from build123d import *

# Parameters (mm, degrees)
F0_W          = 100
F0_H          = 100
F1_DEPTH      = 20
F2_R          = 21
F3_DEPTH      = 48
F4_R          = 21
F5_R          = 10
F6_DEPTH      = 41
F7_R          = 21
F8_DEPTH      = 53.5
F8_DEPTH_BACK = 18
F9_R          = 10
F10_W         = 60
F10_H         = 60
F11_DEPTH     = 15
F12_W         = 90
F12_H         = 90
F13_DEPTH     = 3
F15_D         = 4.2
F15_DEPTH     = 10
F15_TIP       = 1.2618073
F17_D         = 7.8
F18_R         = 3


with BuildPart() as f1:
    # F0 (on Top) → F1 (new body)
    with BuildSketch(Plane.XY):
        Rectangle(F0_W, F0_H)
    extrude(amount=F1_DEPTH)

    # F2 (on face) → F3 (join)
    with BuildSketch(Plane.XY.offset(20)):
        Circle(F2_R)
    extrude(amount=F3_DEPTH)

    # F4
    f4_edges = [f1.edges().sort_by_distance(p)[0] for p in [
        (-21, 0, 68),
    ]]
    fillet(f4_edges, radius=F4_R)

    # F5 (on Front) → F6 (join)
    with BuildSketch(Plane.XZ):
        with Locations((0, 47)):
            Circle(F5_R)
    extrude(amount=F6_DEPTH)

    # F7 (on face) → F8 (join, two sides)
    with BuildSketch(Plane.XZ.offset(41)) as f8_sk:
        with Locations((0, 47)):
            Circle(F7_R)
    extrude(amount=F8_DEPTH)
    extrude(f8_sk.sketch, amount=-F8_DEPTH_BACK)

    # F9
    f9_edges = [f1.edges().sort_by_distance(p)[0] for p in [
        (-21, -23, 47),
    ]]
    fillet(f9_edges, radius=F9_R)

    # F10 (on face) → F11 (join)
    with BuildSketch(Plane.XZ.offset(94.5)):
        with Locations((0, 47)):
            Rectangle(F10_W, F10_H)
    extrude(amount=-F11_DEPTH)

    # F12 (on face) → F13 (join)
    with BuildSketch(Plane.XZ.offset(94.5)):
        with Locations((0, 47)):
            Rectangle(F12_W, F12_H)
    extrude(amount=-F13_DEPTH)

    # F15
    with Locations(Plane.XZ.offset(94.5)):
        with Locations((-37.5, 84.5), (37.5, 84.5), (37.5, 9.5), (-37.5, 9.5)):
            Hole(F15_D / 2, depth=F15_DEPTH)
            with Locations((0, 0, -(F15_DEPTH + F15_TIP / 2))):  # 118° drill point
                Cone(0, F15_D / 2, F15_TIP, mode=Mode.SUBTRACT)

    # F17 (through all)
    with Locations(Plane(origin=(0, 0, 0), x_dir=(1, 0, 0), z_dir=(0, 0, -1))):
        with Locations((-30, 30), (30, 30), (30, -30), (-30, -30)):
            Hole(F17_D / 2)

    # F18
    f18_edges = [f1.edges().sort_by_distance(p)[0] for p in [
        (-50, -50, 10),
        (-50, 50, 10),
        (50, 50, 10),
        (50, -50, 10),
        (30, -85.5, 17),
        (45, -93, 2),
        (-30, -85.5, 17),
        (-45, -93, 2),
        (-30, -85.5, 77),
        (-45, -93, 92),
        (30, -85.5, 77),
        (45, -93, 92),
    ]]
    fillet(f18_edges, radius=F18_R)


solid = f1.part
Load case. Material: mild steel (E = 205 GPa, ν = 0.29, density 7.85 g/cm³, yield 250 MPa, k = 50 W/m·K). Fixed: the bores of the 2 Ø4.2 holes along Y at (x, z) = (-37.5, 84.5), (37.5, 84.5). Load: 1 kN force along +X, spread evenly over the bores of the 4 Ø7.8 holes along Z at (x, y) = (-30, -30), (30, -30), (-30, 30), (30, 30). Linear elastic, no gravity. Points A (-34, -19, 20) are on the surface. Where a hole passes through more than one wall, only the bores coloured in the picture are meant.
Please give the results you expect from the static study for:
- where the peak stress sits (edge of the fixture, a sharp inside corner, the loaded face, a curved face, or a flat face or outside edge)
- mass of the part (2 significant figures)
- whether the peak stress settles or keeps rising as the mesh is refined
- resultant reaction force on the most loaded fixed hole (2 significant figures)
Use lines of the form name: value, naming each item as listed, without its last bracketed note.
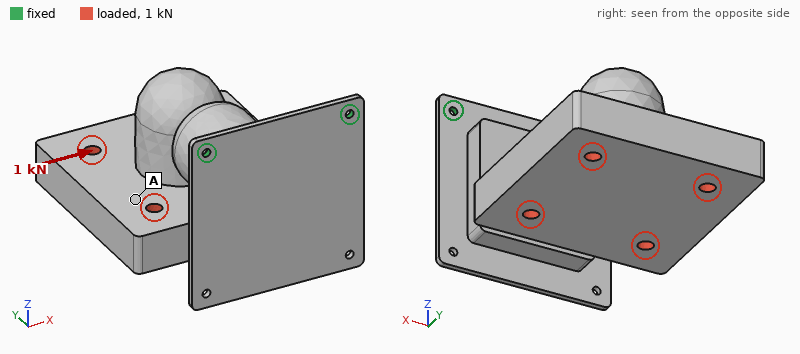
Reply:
where the peak stress sits: edge of the fixture
mass of the part: 3.1 kg
whether the peak stress settles or keeps rising as the mesh is refined: keeps rising
resultant reaction force on the most loaded fixed hole: 1.8 kN
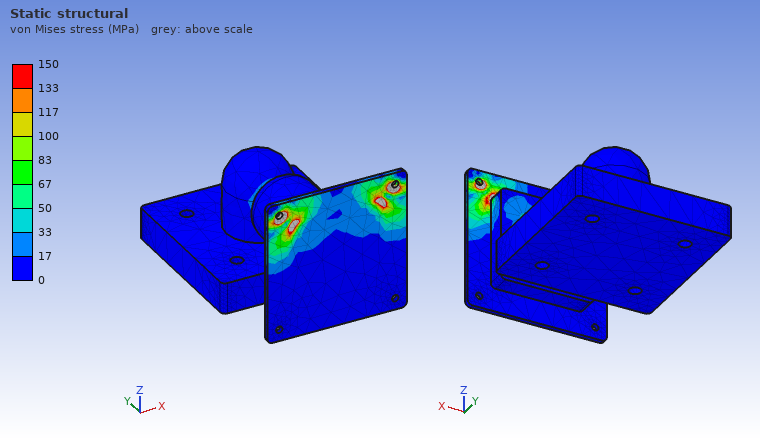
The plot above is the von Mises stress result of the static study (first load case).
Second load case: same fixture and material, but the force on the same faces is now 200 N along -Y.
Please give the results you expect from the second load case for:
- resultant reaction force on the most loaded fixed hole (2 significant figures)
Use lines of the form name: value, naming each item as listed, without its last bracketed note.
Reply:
resultant reaction force on the most loaded fixed hole: 100 N
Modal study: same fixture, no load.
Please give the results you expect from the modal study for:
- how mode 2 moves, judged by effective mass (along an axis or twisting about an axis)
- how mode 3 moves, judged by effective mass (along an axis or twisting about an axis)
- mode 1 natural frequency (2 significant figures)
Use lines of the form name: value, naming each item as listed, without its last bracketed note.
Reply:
how mode 2 moves, judged by effective mass: along X
how mode 3 moves, judged by effective mass: along Y
mode 1 natural frequency: 44 Hz
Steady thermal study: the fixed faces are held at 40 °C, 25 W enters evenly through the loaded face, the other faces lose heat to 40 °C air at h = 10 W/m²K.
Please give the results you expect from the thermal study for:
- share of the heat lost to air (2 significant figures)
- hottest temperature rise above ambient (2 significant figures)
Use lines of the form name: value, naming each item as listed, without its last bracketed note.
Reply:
share of the heat lost to air: 74 %
hottest temperature rise above ambient: 46 K
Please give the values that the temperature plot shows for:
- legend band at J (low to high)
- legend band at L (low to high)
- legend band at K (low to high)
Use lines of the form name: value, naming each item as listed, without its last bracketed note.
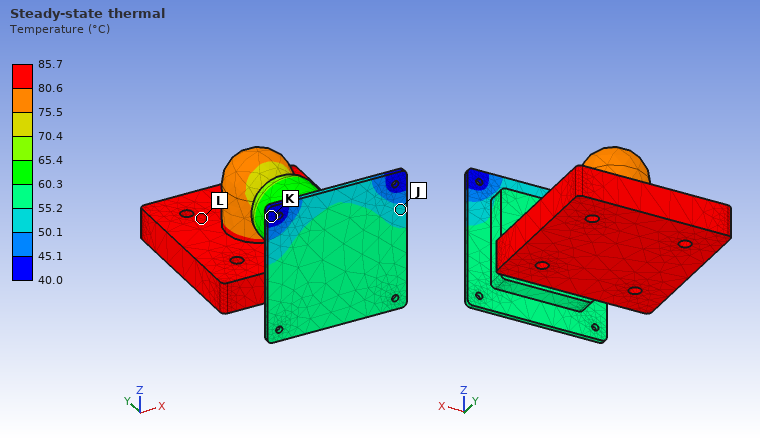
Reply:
legend band at J: 50.1 to 55.2 °C
legend band at L: 80.6 to 85.7 °C
legend band at K: 40.0 to 45.1 °C
